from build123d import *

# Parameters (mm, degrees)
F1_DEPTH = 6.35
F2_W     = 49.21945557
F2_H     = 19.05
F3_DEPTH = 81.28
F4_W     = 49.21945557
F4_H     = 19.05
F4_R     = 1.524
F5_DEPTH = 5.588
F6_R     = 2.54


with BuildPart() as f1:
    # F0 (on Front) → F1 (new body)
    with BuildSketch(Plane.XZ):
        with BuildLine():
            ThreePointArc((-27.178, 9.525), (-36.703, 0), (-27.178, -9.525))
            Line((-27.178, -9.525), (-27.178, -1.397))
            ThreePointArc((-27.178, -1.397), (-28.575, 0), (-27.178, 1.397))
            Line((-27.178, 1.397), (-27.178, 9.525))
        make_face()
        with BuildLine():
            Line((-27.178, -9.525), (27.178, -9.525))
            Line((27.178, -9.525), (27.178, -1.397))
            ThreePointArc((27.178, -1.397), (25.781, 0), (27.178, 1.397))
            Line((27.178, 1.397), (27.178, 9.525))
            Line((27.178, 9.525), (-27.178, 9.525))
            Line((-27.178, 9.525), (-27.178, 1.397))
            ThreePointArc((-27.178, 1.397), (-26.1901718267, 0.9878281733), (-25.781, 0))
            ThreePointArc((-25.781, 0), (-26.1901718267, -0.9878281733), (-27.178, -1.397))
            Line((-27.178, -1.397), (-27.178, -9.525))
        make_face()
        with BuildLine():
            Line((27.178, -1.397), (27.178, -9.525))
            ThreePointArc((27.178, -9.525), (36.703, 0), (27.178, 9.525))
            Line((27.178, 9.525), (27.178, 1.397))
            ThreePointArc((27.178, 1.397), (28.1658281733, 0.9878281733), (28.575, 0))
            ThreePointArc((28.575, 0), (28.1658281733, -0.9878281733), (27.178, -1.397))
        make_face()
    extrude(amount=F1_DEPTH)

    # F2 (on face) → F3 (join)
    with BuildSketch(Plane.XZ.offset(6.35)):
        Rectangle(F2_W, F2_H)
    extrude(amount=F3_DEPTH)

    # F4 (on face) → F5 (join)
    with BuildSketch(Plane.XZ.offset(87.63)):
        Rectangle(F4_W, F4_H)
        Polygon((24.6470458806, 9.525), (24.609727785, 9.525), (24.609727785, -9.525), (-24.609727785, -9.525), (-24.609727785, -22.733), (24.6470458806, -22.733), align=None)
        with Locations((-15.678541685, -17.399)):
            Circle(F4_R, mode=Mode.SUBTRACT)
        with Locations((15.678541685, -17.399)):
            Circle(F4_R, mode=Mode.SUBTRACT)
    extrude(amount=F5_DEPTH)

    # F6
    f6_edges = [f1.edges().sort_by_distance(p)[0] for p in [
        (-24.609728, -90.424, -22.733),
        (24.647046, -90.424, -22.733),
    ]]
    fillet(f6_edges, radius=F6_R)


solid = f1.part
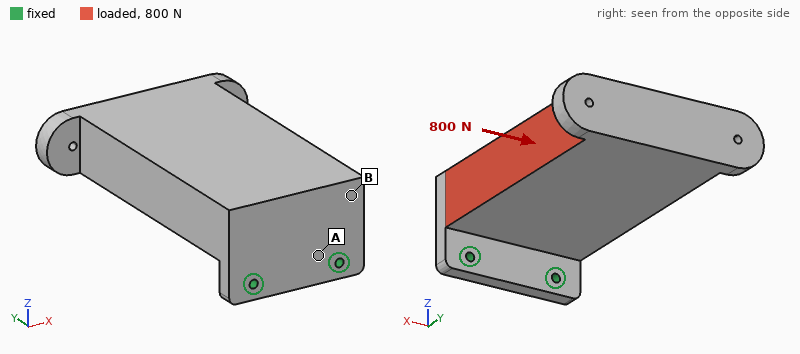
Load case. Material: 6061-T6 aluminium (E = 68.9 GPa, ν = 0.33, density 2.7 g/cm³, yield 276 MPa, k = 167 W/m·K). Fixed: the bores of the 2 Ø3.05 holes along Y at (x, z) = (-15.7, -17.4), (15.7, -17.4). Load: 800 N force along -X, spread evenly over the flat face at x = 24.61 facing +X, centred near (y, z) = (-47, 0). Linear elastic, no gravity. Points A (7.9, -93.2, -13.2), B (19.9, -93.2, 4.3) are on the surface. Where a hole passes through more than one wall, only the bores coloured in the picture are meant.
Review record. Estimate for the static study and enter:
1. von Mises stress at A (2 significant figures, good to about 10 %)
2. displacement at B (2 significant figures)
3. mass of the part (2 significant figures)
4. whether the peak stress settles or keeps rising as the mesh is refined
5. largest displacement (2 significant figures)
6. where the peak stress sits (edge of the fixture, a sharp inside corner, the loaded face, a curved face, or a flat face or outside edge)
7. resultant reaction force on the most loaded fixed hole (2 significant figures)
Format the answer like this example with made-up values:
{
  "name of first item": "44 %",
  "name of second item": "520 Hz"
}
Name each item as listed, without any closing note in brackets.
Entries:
{
  "von Mises stress at A": "11 MPa",
  "displacement at B": "18 µm",
  "mass of the part": "250 g",
  "whether the peak stress settles or keeps rising as the mesh is refined": "keeps rising",
  "largest displacement": "92 µm",
  "where the peak stress sits": "edge of the fixture",
  "resultant reaction force on the most loaded fixed hole": "1.2 kN"
}
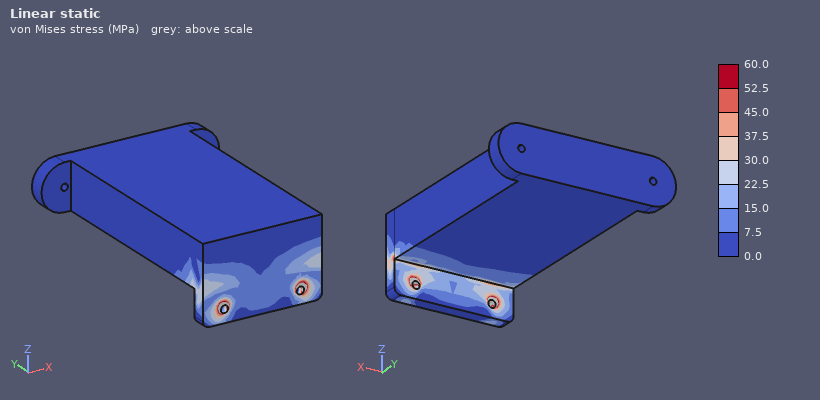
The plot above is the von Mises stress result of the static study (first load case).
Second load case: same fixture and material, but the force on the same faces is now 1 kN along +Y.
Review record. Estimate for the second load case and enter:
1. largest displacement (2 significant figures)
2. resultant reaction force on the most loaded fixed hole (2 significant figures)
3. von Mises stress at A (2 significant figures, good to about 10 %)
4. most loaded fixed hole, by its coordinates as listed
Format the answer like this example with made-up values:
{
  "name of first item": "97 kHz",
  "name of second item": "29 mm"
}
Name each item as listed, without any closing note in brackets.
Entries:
{
  "largest displacement": "0.36 mm",
  "resultant reaction force on the most loaded fixed hole": "1.2 kN",
  "von Mises stress at A": "33 MPa",
  "most loaded fixed hole, by its coordinates as listed": "(15.7, -17.4)"
}
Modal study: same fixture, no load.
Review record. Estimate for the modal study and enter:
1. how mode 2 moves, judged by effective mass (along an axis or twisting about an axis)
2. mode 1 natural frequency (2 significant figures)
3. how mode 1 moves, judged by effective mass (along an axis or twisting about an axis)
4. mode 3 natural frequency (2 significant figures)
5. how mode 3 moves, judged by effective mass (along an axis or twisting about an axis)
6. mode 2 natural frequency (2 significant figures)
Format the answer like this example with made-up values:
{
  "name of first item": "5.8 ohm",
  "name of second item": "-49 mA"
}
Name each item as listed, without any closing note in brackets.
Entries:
{
  "how mode 2 moves, judged by effective mass": "along X",
  "mode 1 natural frequency": "350 Hz",
  "how mode 1 moves, judged by effective mass": "along Z",
  "mode 3 natural frequency": "3700 Hz",
  "how mode 3 moves, judged by effective mass": "along Y",
  "mode 2 natural frequency": "1100 Hz"
}
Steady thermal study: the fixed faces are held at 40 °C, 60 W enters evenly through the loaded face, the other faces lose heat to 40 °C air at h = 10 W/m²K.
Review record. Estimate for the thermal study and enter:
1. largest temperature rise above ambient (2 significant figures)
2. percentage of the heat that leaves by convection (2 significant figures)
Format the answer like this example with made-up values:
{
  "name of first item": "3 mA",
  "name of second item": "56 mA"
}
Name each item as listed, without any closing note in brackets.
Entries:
{
  "largest temperature rise above ambient": "38 K",
  "percentage of the heat that leaves by convection": "7.0 %"
}
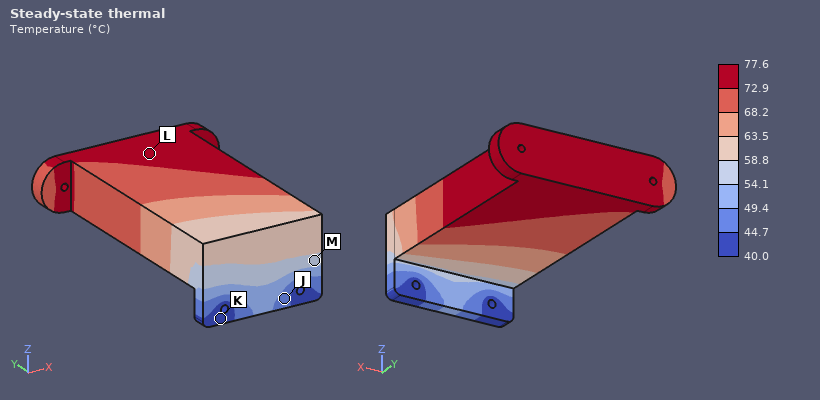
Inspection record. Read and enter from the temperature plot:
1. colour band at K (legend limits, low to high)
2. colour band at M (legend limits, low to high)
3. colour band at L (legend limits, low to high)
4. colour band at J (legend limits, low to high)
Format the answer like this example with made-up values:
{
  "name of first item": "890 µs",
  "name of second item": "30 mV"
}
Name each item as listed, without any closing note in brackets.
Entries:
{
  "colour band at K": "40.0 to 44.7 °C",
  "colour band at M": "54.1 to 58.8 °C",
  "colour band at L": "72.9 to 77.6 °C",
  "colour band at J": "44.7 to 49.4 °C"
}
